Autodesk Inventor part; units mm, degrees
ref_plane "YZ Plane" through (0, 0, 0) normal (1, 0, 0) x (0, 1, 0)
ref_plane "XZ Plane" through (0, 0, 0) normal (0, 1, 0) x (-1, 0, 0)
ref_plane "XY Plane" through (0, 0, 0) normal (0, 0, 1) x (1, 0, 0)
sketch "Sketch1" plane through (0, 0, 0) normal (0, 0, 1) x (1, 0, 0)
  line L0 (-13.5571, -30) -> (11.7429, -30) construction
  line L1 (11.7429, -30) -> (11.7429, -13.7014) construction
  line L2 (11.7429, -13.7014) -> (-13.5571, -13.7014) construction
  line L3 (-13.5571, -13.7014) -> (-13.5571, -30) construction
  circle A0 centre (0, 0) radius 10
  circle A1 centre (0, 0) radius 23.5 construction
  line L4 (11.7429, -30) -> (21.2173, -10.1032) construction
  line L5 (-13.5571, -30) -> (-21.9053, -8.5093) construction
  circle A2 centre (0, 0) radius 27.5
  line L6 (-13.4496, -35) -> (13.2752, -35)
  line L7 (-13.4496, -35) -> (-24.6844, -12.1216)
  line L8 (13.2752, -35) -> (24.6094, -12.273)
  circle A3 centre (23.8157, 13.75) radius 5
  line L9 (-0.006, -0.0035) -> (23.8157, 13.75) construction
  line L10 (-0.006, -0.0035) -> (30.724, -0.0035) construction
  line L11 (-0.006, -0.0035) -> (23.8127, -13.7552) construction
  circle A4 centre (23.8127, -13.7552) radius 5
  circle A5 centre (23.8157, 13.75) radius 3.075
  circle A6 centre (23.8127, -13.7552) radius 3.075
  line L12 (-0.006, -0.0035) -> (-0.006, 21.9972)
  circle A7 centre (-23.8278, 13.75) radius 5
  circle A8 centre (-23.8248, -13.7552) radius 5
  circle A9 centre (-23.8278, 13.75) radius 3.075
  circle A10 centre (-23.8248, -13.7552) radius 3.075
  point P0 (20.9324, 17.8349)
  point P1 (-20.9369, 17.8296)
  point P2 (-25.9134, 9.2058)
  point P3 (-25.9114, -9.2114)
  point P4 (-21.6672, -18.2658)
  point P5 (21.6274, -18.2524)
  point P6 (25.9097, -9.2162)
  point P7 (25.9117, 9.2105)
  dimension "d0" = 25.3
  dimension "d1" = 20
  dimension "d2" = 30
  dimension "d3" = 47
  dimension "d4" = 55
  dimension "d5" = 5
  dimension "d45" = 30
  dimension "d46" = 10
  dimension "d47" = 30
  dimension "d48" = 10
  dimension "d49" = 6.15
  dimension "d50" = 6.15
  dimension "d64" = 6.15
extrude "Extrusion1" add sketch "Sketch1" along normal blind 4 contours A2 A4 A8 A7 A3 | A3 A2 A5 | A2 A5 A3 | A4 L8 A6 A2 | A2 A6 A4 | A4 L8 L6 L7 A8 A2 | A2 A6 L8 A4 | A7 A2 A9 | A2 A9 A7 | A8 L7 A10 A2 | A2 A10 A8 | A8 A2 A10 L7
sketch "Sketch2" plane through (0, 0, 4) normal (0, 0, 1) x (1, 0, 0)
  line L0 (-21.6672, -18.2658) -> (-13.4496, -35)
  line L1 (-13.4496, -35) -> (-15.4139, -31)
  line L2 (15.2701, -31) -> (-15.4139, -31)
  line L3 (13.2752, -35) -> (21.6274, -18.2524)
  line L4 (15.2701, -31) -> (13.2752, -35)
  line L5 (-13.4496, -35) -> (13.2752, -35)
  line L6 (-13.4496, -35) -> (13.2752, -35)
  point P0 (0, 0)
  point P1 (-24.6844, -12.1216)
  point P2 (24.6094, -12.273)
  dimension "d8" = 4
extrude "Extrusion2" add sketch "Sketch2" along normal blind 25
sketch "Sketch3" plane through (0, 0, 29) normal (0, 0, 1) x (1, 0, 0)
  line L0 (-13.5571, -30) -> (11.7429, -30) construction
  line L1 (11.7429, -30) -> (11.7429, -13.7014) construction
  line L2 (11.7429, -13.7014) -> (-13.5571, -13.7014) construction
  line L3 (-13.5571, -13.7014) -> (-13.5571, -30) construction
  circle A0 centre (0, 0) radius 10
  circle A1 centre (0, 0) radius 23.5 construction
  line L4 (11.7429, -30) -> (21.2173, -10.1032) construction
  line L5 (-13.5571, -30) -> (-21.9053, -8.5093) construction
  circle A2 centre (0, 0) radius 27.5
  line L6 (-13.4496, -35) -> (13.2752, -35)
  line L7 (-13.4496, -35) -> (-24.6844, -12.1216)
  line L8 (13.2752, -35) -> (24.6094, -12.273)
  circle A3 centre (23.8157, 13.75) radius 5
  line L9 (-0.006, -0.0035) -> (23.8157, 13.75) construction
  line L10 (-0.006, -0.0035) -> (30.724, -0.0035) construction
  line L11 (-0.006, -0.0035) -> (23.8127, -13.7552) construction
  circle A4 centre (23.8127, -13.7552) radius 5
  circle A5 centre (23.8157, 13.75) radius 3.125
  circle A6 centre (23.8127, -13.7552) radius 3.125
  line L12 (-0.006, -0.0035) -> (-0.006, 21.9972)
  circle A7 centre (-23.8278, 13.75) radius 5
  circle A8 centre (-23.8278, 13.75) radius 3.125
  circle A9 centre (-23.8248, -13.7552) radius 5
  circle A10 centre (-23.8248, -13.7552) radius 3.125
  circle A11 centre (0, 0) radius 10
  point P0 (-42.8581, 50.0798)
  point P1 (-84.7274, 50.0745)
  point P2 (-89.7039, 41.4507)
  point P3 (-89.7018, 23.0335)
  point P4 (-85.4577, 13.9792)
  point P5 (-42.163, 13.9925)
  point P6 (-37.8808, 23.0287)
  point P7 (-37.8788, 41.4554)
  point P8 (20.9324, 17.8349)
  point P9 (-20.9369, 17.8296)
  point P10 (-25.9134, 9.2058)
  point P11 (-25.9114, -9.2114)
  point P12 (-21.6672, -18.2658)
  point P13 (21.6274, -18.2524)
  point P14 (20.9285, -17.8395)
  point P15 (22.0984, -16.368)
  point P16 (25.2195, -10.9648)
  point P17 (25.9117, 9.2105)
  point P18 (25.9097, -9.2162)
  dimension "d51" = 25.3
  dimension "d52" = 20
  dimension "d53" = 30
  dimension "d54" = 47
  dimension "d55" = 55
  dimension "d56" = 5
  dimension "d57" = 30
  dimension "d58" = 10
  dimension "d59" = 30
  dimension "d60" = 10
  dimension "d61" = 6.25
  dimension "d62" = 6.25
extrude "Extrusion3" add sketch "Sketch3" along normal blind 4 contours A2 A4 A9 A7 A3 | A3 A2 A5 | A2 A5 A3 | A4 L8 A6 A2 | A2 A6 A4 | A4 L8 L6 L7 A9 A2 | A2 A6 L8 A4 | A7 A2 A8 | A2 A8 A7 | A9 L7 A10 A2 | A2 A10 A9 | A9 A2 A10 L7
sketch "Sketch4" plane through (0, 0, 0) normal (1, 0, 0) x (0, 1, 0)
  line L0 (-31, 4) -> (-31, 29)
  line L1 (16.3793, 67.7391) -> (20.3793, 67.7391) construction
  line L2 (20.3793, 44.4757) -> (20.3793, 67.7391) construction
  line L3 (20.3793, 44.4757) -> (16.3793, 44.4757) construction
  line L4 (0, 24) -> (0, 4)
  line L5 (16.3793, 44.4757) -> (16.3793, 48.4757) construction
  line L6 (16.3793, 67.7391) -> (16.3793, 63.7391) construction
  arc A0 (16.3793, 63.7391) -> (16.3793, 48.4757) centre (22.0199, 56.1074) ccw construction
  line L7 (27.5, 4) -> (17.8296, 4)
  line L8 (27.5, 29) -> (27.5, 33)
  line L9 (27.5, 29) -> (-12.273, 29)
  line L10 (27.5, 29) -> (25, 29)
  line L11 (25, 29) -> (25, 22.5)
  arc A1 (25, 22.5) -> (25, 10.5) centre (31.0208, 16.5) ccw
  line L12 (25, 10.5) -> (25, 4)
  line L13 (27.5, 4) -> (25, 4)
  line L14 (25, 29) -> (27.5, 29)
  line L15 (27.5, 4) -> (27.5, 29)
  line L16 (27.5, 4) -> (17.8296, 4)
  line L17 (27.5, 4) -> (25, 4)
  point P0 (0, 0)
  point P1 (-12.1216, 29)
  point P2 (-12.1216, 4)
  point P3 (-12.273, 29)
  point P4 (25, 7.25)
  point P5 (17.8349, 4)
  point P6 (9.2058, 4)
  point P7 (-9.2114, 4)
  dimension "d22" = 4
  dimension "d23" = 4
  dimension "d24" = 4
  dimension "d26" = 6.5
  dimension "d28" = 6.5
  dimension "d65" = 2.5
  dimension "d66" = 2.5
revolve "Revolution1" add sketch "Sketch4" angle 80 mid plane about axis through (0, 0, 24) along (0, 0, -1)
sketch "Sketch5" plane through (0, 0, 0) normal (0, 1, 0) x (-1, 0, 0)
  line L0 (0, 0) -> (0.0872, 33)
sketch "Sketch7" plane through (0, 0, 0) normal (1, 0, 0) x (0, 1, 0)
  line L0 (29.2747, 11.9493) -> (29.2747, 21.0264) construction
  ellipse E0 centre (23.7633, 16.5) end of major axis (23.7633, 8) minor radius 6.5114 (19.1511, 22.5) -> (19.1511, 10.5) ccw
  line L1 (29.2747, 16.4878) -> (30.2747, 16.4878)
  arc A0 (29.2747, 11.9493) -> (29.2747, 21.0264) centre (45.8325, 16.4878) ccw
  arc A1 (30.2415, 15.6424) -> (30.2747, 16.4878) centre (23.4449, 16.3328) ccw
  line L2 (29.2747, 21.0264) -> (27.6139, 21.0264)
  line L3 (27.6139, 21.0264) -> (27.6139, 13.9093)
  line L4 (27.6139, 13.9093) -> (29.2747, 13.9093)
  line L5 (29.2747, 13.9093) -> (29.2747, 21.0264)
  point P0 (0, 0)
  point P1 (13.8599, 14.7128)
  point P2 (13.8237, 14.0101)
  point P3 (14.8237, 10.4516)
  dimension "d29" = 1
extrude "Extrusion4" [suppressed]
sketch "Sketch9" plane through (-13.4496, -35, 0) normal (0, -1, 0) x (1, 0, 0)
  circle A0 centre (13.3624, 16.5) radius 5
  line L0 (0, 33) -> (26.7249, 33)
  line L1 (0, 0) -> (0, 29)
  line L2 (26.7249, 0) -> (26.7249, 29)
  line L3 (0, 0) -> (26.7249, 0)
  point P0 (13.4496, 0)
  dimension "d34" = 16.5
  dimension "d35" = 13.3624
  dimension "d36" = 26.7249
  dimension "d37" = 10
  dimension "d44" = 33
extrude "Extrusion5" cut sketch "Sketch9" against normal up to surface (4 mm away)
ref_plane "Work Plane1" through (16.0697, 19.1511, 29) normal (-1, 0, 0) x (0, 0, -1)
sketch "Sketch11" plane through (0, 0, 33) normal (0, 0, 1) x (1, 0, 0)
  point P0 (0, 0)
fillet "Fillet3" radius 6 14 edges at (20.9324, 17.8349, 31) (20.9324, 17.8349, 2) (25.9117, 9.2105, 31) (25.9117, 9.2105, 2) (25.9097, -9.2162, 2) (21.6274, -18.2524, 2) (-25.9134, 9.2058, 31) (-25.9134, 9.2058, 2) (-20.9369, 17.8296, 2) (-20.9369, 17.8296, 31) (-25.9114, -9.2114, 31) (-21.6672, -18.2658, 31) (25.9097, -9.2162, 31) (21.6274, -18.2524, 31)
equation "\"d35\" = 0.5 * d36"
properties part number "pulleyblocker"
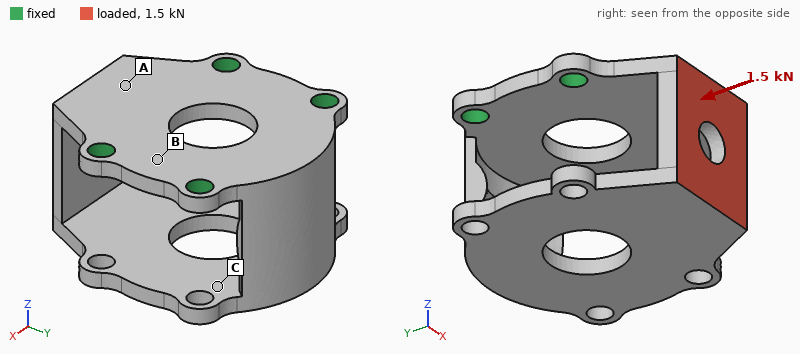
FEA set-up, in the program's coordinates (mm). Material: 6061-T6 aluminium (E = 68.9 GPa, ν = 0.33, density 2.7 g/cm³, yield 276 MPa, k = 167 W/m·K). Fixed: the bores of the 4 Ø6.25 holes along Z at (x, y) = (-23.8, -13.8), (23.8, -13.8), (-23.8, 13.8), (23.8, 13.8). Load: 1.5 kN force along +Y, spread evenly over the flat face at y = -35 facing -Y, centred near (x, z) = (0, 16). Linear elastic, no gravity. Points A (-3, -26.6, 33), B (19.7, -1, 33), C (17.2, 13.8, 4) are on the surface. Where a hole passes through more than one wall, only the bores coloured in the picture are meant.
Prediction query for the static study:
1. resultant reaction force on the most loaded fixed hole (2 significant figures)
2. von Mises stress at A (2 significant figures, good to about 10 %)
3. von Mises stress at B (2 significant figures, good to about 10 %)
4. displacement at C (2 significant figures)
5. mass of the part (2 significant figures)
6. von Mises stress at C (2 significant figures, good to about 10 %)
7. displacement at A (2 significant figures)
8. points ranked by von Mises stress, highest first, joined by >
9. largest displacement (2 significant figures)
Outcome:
540 N
66 MPa
11 MPa
0.32 mm
68 g
39 MPa
0.083 mm
A > C > B
0.38 mm
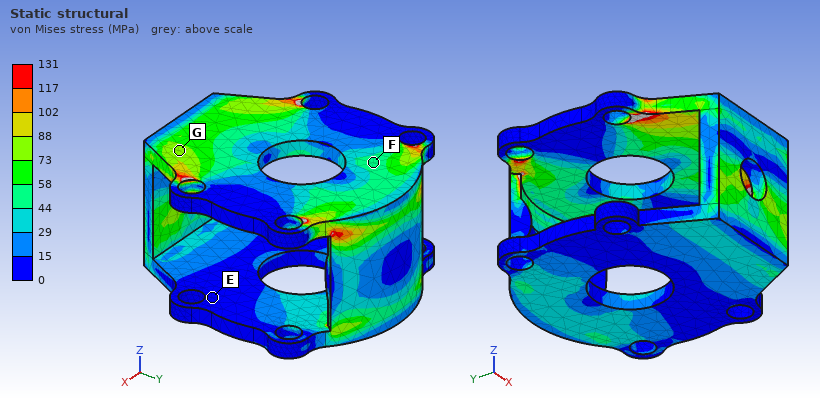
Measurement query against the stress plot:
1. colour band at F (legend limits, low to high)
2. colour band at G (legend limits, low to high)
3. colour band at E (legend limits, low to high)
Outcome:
44 to 58 MPa
73 to 88 MPa
0 to 15 MPa
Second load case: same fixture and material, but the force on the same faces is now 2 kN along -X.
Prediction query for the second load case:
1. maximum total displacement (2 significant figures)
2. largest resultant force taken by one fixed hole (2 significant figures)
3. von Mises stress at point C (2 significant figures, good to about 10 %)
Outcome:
0.32 mm
1.4 kN
31 MPa
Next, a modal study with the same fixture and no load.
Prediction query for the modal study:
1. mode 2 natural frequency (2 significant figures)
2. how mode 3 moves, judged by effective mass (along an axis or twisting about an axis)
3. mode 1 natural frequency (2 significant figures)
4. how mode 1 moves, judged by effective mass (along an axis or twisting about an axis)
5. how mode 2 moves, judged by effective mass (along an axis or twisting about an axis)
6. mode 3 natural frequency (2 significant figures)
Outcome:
2300 Hz
along Z
1300 Hz
along Y
along X
2700 Hz
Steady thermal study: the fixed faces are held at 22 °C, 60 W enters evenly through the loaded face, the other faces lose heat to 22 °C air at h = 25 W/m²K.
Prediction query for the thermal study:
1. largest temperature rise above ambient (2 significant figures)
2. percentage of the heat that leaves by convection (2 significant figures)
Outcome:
66 K
17 %
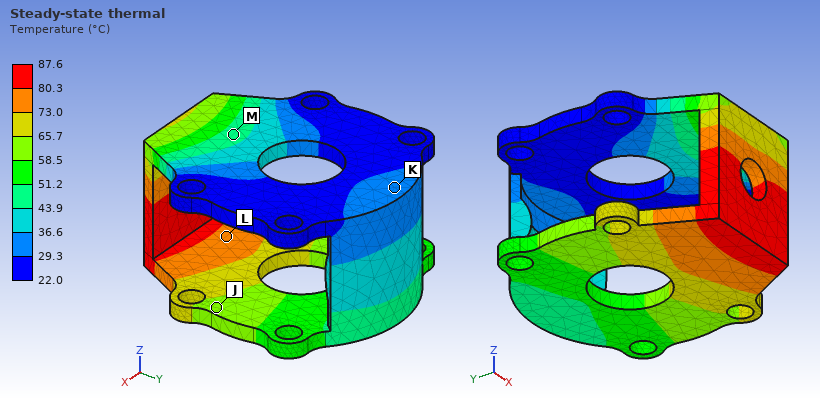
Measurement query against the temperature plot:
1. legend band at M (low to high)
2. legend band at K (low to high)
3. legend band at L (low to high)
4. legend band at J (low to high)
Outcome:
43.9 to 51.2 °C
29.3 to 36.6 °C
73.0 to 80.3 °C
58.5 to 65.7 °C
